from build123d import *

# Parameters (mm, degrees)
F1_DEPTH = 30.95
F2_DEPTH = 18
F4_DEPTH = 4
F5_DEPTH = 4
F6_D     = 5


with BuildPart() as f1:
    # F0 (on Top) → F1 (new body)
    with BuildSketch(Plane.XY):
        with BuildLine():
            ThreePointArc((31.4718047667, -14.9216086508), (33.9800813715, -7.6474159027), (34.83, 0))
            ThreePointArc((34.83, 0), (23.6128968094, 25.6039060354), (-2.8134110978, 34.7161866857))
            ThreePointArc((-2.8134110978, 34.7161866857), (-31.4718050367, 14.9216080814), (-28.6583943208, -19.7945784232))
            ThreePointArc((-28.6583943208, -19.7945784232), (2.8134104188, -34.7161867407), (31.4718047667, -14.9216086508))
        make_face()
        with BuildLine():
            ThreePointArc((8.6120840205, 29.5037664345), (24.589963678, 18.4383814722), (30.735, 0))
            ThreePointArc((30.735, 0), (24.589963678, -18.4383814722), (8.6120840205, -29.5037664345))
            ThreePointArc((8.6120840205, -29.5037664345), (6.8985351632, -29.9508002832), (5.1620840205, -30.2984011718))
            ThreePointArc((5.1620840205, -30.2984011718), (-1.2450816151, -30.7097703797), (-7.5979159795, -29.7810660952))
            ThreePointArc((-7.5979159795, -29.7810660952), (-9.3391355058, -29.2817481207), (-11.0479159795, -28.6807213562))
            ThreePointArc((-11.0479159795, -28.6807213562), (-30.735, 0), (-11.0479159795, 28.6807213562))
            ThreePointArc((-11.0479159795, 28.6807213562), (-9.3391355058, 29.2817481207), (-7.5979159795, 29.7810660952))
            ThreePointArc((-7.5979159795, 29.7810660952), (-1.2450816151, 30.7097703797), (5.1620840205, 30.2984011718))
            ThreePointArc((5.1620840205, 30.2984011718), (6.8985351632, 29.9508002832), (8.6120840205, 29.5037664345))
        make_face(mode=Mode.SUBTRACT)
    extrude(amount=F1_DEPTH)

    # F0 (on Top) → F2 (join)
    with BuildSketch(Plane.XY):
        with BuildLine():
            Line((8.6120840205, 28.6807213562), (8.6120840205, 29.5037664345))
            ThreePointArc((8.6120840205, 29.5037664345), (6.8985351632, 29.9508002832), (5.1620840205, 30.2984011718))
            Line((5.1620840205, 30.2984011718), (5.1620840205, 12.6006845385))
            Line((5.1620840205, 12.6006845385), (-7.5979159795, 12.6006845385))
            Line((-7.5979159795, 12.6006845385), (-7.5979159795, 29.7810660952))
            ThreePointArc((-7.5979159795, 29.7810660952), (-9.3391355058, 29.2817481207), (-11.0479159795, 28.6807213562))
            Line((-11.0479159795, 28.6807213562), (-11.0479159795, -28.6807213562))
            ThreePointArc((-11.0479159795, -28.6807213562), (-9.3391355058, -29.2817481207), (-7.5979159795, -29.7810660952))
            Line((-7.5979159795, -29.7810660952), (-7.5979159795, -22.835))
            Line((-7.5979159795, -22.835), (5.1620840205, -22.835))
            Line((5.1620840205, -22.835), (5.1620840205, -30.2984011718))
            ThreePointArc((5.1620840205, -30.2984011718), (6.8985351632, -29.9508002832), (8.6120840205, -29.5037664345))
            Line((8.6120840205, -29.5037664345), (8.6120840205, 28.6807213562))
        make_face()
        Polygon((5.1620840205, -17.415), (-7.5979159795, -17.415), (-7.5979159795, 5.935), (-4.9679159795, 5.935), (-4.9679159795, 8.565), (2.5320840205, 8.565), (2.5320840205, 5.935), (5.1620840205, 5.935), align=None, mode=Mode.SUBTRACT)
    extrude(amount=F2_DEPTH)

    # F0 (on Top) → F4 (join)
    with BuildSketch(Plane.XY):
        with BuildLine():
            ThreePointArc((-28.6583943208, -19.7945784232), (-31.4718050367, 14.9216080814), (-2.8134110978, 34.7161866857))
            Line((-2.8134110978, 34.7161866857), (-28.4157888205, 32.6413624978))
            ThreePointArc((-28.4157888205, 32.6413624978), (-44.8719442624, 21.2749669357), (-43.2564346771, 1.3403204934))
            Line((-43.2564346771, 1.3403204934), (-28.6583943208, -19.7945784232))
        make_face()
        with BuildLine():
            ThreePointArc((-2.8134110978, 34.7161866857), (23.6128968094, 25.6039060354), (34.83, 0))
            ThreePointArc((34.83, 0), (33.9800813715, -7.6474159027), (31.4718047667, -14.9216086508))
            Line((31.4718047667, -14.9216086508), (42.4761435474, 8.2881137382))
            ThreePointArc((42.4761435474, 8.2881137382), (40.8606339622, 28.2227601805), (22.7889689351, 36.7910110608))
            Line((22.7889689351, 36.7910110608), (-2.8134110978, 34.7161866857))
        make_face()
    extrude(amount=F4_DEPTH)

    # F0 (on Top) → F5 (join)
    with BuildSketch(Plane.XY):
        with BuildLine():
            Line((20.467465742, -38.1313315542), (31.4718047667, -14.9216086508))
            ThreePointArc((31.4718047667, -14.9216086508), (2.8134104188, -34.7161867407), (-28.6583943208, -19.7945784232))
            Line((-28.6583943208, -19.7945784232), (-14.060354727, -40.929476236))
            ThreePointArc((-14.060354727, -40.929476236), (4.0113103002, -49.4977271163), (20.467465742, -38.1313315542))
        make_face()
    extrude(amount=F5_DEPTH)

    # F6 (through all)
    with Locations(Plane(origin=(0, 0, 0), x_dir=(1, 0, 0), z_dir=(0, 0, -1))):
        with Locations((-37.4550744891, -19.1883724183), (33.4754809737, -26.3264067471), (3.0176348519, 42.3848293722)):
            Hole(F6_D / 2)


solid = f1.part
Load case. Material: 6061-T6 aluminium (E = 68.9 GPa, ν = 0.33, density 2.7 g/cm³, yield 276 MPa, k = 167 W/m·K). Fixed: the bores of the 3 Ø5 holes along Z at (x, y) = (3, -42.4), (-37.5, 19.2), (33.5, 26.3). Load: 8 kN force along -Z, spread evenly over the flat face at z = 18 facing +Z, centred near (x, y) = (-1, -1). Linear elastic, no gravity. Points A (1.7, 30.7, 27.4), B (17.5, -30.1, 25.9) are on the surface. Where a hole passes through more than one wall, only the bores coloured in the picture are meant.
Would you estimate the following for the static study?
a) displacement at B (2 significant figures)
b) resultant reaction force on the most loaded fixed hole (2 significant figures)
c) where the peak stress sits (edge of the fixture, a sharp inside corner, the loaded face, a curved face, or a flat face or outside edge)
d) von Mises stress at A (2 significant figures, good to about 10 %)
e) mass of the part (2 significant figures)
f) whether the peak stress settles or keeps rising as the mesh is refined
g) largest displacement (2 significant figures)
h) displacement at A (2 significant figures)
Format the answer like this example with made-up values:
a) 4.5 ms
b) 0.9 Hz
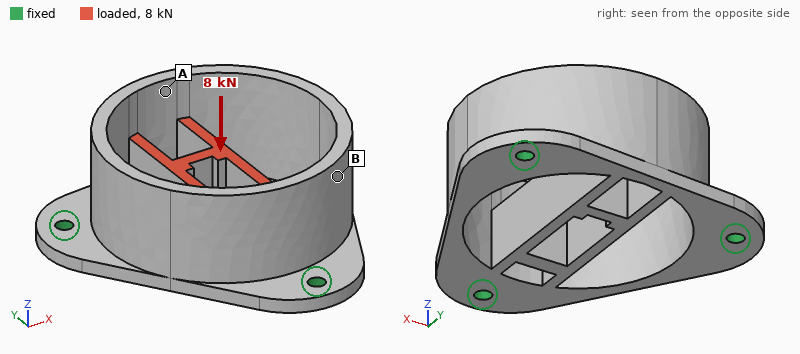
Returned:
a) 0.062 mm
b) 3.2 kN
c) edge of the fixture
d) 52 MPa
e) 110 g
f) keeps rising
g) 0.15 mm
h) 0.070 mm
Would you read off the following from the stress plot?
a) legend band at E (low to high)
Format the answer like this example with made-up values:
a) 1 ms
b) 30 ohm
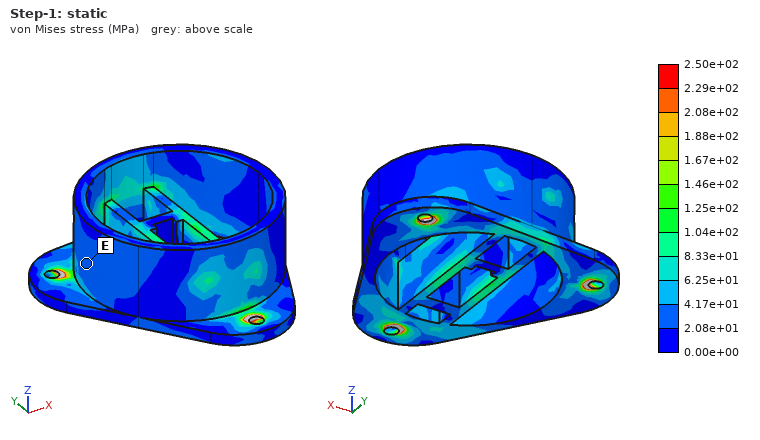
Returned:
a) 2.08e+01 to 4.17e+01 MPa
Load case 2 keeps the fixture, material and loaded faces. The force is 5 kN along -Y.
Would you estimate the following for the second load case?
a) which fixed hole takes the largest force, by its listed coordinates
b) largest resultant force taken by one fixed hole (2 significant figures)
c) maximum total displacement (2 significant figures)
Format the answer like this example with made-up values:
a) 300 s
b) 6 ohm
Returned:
a) (3, -42.4)
b) 3.4 kN
c) 74 µm
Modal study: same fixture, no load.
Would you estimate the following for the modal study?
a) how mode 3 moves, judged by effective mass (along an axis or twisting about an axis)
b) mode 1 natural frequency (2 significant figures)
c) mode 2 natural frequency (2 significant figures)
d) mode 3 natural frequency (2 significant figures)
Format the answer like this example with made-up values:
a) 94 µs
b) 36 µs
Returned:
a) along Z
b) 3600 Hz
c) 5100 Hz
d) 5300 Hz
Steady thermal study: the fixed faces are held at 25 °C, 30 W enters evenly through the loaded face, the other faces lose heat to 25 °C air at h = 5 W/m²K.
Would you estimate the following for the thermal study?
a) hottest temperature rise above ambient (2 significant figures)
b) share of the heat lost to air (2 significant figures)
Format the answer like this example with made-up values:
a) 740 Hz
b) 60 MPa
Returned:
a) 23 K
b) 3.8 %
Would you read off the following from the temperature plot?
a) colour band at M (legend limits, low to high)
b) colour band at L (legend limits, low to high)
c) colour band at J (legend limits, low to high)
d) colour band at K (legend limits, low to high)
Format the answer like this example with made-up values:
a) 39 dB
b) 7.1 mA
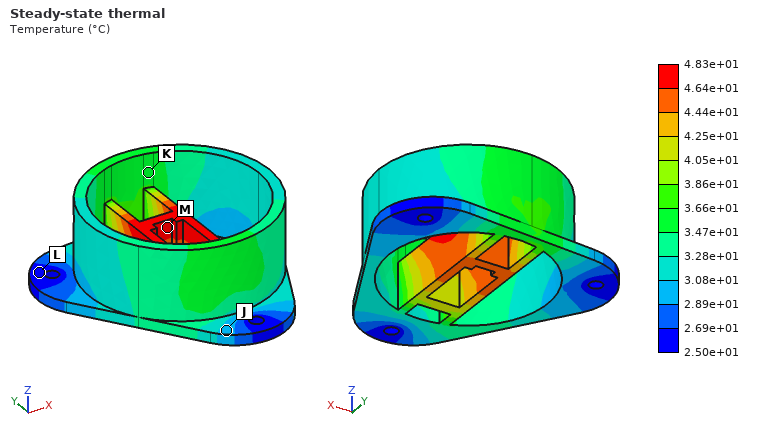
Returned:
a) 4.64e+01 to 4.83e+01 °C
b) 2.50e+01 to 2.69e+01 °C
c) 2.89e+01 to 3.08e+01 °C
d) 3.47e+01 to 3.66e+01 °C
